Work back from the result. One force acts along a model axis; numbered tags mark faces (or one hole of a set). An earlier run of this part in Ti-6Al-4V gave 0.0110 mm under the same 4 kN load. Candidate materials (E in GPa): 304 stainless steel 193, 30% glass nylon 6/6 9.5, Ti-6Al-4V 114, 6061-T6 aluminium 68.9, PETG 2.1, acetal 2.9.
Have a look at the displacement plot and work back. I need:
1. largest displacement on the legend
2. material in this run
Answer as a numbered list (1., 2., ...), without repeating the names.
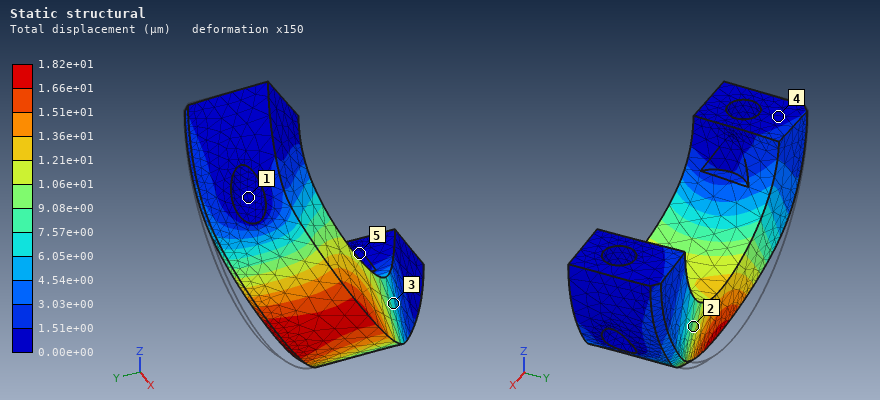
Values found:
1. 1.82e+01 µm
2. 6061-T6 aluminium
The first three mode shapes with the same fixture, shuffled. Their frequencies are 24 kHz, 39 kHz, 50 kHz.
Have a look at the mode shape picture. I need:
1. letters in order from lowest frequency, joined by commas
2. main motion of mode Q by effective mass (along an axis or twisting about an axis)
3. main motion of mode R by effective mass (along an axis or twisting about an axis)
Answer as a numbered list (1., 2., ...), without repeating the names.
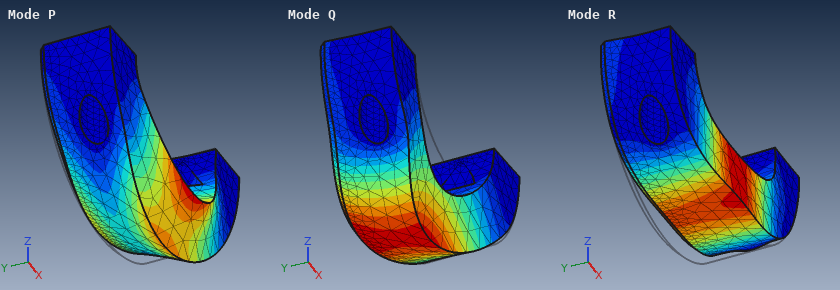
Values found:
1. Q, R, P
2. along Y
3. along Z
